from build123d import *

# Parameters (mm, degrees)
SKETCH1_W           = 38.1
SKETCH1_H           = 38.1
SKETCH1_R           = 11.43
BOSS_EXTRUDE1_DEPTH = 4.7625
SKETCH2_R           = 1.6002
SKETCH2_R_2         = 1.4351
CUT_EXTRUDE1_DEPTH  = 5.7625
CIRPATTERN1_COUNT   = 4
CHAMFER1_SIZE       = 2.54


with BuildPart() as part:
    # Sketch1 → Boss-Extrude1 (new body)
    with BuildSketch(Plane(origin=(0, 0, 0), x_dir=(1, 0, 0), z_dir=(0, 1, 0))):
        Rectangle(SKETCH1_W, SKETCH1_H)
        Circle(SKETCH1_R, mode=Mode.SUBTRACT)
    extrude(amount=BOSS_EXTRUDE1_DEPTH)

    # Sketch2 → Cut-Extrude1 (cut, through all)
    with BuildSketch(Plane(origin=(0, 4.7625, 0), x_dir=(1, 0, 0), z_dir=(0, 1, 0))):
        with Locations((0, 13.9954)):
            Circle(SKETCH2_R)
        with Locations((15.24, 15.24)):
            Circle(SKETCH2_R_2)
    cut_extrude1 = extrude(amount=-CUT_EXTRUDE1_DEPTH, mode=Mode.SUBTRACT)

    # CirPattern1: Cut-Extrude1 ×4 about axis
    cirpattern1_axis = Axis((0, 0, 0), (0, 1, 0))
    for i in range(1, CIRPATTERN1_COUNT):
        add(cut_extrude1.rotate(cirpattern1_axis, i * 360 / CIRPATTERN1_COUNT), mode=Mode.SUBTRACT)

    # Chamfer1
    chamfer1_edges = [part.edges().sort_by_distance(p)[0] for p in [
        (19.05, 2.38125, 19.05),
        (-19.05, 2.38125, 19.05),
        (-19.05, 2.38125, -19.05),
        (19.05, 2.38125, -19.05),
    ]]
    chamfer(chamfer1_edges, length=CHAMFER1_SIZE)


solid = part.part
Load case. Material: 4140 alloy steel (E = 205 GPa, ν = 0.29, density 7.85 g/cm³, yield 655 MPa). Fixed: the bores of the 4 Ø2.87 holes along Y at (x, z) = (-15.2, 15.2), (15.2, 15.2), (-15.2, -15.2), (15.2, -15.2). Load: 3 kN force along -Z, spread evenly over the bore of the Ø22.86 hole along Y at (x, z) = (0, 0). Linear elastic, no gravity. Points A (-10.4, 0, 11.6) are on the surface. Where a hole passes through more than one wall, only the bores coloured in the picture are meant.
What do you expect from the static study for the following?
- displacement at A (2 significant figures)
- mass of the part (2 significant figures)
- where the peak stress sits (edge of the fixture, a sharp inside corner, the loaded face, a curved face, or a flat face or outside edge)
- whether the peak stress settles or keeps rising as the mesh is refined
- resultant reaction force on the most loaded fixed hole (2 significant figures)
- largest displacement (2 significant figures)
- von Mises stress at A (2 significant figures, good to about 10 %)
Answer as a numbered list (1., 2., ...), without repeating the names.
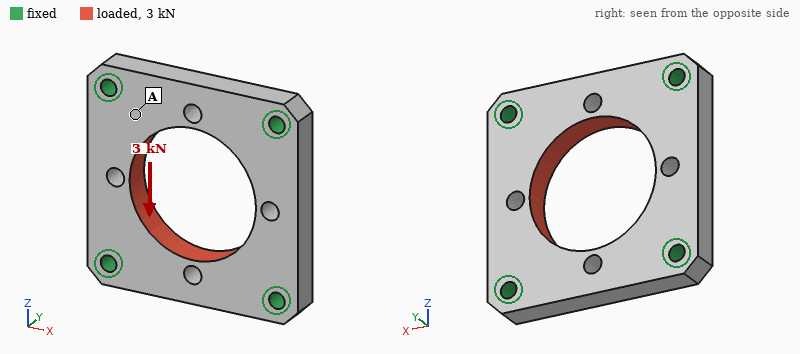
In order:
1. 1.1 µm
2. 36 g
3. edge of the fixture
4. keeps rising
5. 770 N
6. 3.1 µm
7. 14 MPa
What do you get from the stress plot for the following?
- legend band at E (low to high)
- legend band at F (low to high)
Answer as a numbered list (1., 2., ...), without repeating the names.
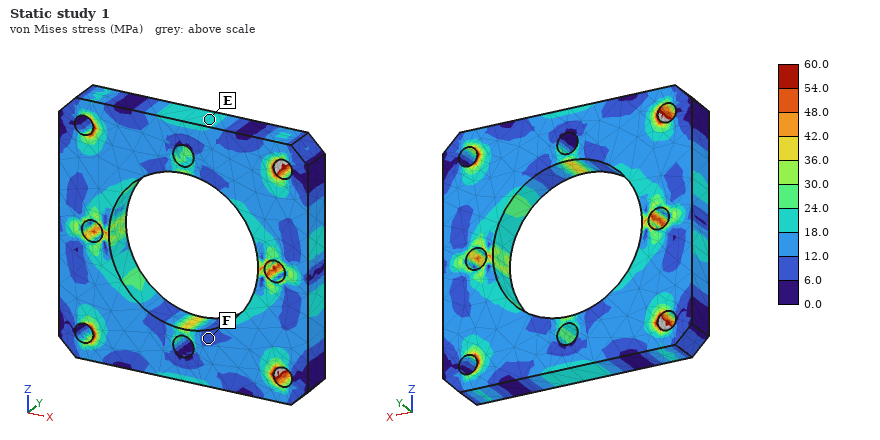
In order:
1. 18.0 to 24.0 MPa
2. 6.0 to 12.0 MPa
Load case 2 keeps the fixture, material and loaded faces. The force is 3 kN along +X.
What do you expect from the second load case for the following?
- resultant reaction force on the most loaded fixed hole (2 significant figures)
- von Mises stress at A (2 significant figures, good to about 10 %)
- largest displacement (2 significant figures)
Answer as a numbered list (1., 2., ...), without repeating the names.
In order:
1. 770 N
2. 14 MPa
3. 3.1 µm
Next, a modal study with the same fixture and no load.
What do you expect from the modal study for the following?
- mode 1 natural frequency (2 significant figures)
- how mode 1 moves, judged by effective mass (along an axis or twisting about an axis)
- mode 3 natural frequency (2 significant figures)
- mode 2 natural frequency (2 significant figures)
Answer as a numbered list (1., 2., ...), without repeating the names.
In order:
1. 23 kHz
2. along Y
3. 25 kHz
4. 25 kHz
